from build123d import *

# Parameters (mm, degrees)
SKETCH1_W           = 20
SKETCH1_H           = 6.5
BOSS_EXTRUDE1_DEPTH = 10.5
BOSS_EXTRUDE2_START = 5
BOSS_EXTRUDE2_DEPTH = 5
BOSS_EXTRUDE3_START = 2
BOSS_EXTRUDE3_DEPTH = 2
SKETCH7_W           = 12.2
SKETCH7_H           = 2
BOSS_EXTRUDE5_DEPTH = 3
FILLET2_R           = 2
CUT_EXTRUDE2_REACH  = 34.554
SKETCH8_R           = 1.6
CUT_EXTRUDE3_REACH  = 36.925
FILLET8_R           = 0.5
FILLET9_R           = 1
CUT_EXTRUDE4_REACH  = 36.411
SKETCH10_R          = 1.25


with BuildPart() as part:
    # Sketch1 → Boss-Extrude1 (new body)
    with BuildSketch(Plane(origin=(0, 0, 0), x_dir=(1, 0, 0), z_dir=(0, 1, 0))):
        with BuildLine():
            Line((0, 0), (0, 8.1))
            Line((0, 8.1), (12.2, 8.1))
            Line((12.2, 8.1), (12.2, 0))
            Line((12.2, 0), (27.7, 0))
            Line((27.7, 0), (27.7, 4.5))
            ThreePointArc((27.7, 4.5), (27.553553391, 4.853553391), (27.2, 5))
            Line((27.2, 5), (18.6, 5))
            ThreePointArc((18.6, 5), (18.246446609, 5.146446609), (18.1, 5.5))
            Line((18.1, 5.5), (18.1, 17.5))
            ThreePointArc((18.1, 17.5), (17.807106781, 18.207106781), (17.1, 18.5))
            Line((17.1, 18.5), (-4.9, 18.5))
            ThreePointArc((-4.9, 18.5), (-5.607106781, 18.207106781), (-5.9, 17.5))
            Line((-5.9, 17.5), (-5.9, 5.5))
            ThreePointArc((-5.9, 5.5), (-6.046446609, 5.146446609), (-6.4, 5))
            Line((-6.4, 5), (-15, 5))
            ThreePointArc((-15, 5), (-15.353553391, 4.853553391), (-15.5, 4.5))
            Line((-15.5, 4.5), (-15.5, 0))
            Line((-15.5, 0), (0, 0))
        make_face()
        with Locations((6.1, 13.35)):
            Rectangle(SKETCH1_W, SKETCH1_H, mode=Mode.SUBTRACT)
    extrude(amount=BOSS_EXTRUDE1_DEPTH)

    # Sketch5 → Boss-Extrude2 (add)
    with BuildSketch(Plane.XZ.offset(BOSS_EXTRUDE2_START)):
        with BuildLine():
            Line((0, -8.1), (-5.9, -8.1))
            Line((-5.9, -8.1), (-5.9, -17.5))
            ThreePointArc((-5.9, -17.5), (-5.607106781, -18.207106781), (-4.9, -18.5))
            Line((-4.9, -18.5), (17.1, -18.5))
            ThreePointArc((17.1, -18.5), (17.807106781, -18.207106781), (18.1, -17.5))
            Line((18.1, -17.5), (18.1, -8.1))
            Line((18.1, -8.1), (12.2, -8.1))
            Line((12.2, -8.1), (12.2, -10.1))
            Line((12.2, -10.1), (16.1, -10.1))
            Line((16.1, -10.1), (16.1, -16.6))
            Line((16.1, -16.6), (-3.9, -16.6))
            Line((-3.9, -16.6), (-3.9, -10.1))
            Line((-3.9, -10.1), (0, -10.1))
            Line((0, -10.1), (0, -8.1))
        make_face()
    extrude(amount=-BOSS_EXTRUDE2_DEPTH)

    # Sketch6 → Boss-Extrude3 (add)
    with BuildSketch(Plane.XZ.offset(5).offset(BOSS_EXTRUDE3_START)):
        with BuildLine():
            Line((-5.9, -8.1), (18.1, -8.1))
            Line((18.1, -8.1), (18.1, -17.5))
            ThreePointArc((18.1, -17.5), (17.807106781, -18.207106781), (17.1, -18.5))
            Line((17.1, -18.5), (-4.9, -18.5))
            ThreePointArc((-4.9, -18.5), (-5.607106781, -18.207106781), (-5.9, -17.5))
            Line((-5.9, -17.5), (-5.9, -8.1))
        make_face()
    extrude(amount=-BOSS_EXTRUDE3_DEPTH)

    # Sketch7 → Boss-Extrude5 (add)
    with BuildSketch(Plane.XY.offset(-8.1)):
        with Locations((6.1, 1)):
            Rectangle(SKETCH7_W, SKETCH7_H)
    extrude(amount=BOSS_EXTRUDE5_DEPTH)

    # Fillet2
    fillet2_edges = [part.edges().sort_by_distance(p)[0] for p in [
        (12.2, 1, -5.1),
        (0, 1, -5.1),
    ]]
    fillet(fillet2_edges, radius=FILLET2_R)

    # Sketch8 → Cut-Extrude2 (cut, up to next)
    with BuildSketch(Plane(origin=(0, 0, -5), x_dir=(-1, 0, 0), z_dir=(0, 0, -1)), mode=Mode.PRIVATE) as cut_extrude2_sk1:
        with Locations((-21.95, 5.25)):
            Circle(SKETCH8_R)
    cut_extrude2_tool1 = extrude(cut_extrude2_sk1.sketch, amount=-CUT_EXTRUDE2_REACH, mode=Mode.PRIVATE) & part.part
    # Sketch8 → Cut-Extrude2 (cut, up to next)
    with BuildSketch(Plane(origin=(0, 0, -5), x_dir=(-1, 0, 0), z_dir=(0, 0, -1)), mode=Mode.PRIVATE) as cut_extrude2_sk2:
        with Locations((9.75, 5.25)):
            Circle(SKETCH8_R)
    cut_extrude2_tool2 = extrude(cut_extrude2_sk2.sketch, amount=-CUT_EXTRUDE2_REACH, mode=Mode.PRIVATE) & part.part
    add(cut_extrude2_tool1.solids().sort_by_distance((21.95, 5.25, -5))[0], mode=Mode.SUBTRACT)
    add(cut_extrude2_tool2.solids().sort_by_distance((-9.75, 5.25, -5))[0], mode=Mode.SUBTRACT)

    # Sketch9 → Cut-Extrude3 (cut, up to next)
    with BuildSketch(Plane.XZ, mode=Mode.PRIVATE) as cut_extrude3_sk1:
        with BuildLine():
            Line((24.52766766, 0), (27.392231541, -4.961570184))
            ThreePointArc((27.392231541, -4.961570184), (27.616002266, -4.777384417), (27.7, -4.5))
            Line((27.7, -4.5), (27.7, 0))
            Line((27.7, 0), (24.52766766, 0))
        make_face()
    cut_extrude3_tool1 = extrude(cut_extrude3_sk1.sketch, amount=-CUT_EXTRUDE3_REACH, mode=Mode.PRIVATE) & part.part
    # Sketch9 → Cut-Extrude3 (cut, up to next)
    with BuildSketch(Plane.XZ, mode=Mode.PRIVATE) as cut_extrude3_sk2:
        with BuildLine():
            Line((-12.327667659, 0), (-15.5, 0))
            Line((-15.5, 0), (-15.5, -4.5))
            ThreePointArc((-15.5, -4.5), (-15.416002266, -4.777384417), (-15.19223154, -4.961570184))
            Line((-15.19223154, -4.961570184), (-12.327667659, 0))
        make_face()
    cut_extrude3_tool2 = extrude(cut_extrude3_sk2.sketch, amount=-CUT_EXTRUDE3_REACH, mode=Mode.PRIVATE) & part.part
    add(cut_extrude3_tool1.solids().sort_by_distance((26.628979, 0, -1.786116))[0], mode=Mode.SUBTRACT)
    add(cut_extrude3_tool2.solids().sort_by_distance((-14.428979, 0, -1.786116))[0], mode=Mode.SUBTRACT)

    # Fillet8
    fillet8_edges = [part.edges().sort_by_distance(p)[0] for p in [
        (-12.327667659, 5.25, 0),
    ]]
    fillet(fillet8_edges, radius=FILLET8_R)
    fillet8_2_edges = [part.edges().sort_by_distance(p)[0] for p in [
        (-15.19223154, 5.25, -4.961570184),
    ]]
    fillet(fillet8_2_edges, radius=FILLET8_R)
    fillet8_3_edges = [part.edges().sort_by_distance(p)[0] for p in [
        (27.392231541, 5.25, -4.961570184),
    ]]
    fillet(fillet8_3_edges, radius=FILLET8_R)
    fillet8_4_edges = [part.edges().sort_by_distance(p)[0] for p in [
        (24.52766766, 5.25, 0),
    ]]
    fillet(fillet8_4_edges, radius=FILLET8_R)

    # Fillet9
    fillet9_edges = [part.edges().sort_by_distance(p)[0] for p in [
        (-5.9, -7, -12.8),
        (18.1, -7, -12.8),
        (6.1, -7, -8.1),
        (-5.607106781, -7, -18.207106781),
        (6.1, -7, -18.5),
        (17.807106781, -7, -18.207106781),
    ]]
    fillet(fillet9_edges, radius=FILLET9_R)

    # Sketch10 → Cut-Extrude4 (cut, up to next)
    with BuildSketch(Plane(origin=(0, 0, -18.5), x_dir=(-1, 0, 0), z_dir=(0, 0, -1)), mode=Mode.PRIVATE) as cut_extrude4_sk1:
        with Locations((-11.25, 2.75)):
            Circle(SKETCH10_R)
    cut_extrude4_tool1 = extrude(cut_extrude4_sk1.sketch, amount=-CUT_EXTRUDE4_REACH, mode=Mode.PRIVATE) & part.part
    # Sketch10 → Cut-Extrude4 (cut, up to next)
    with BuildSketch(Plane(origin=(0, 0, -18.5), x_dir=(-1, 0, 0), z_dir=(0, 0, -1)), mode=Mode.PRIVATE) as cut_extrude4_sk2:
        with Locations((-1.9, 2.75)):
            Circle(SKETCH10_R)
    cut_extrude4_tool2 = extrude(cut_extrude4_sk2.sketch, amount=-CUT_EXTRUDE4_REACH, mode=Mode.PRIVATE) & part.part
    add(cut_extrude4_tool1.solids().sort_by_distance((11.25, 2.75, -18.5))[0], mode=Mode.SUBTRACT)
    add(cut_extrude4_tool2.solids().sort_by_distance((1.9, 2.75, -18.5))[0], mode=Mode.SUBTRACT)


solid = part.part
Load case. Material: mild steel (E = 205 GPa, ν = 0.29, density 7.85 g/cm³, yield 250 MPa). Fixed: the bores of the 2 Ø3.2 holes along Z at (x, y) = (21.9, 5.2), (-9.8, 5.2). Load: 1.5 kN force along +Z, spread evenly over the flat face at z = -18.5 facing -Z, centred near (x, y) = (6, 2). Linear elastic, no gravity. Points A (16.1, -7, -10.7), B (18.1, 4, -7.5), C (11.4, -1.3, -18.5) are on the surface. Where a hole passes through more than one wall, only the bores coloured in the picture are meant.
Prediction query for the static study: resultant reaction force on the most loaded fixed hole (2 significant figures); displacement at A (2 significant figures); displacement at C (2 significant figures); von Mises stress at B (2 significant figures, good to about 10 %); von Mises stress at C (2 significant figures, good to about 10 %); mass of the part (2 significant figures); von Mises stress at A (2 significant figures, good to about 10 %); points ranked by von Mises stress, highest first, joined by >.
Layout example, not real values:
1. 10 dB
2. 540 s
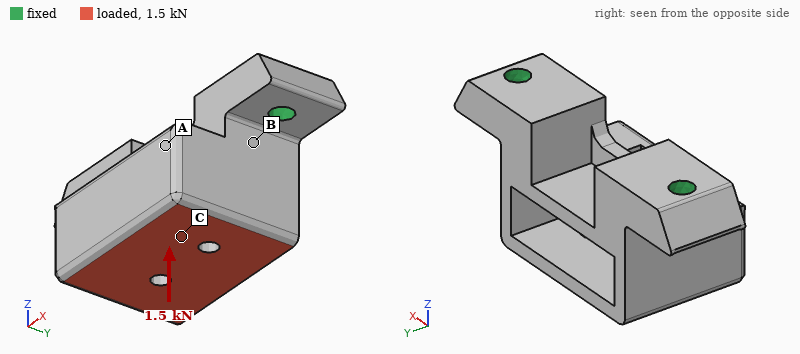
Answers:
1. 770 N
2. 13 µm
3. 17 µm
4. 49 MPa
5. 81 MPa
6. 32 g
7. 19 MPa
8. C > B > A
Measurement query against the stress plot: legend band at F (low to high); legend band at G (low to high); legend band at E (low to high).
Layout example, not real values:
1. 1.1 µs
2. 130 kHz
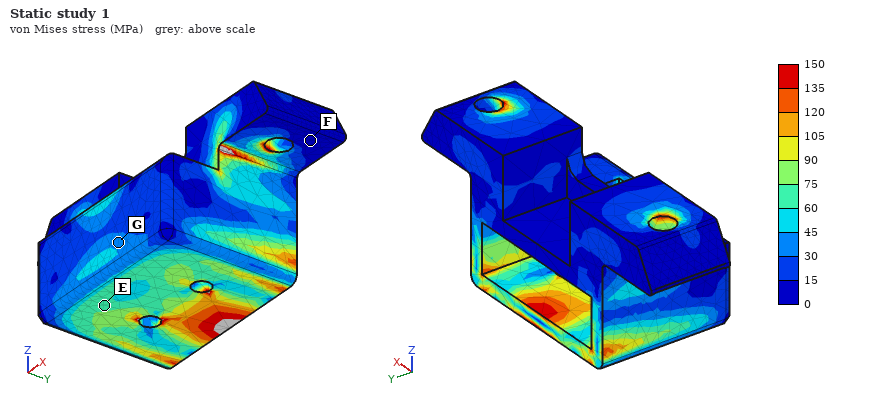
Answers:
1. 0 to 15 MPa
2. 30 to 45 MPa
3. 60 to 75 MPa
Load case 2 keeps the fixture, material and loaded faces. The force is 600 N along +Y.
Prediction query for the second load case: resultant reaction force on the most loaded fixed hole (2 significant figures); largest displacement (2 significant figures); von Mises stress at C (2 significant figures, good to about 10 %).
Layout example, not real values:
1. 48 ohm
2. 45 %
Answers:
1. 300 N
2. 26 µm
3. 15 MPa
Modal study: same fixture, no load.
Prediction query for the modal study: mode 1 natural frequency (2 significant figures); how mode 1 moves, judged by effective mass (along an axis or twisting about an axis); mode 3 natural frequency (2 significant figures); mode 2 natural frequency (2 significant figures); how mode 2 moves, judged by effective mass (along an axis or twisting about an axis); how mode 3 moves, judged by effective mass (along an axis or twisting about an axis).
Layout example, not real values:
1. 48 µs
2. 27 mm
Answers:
1. 7800 Hz
2. along Y
3. 16 kHz
4. 11 kHz
5. along X
6. along X
